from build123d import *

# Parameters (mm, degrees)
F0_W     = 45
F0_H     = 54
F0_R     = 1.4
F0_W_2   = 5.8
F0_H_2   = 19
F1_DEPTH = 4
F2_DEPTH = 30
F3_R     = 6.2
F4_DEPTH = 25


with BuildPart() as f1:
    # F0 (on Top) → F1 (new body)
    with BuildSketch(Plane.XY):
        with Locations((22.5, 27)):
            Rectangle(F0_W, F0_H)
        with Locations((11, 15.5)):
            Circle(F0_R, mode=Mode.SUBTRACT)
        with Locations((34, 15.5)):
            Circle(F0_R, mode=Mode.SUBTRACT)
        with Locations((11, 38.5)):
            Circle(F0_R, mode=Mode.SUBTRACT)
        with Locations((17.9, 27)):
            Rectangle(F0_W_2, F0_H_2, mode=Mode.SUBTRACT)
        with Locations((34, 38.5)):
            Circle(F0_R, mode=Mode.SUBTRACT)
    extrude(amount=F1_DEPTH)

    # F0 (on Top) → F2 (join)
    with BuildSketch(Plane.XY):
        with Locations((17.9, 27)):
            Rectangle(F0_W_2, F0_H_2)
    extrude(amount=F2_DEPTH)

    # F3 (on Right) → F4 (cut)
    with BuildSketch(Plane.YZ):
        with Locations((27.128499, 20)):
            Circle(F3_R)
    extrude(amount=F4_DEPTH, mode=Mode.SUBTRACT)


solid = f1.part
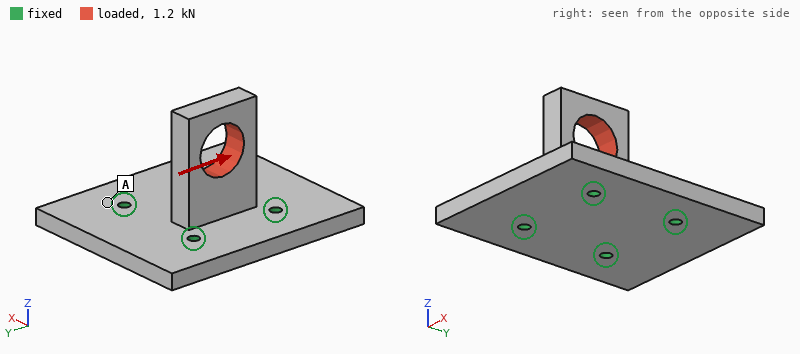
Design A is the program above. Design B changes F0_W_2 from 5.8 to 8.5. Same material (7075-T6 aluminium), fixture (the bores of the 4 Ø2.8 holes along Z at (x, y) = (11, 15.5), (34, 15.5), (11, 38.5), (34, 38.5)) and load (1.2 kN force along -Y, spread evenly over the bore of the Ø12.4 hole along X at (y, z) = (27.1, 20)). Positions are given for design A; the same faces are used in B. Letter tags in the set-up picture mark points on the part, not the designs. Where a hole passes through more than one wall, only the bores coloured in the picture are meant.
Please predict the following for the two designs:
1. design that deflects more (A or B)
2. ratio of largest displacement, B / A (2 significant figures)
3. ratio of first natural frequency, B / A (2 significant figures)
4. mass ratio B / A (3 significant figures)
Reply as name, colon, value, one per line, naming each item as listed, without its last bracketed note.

design that deflects more: A
ratio of largest displacement, B / A: 0.73
ratio of first natural frequency, B / A: 1.2
mass ratio B / A: 1.09
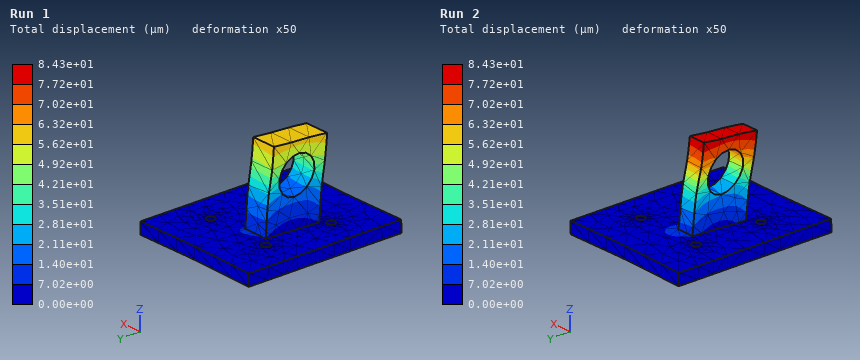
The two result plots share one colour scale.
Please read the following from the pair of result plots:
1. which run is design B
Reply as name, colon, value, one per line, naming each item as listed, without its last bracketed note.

which run is design B: Run 1
